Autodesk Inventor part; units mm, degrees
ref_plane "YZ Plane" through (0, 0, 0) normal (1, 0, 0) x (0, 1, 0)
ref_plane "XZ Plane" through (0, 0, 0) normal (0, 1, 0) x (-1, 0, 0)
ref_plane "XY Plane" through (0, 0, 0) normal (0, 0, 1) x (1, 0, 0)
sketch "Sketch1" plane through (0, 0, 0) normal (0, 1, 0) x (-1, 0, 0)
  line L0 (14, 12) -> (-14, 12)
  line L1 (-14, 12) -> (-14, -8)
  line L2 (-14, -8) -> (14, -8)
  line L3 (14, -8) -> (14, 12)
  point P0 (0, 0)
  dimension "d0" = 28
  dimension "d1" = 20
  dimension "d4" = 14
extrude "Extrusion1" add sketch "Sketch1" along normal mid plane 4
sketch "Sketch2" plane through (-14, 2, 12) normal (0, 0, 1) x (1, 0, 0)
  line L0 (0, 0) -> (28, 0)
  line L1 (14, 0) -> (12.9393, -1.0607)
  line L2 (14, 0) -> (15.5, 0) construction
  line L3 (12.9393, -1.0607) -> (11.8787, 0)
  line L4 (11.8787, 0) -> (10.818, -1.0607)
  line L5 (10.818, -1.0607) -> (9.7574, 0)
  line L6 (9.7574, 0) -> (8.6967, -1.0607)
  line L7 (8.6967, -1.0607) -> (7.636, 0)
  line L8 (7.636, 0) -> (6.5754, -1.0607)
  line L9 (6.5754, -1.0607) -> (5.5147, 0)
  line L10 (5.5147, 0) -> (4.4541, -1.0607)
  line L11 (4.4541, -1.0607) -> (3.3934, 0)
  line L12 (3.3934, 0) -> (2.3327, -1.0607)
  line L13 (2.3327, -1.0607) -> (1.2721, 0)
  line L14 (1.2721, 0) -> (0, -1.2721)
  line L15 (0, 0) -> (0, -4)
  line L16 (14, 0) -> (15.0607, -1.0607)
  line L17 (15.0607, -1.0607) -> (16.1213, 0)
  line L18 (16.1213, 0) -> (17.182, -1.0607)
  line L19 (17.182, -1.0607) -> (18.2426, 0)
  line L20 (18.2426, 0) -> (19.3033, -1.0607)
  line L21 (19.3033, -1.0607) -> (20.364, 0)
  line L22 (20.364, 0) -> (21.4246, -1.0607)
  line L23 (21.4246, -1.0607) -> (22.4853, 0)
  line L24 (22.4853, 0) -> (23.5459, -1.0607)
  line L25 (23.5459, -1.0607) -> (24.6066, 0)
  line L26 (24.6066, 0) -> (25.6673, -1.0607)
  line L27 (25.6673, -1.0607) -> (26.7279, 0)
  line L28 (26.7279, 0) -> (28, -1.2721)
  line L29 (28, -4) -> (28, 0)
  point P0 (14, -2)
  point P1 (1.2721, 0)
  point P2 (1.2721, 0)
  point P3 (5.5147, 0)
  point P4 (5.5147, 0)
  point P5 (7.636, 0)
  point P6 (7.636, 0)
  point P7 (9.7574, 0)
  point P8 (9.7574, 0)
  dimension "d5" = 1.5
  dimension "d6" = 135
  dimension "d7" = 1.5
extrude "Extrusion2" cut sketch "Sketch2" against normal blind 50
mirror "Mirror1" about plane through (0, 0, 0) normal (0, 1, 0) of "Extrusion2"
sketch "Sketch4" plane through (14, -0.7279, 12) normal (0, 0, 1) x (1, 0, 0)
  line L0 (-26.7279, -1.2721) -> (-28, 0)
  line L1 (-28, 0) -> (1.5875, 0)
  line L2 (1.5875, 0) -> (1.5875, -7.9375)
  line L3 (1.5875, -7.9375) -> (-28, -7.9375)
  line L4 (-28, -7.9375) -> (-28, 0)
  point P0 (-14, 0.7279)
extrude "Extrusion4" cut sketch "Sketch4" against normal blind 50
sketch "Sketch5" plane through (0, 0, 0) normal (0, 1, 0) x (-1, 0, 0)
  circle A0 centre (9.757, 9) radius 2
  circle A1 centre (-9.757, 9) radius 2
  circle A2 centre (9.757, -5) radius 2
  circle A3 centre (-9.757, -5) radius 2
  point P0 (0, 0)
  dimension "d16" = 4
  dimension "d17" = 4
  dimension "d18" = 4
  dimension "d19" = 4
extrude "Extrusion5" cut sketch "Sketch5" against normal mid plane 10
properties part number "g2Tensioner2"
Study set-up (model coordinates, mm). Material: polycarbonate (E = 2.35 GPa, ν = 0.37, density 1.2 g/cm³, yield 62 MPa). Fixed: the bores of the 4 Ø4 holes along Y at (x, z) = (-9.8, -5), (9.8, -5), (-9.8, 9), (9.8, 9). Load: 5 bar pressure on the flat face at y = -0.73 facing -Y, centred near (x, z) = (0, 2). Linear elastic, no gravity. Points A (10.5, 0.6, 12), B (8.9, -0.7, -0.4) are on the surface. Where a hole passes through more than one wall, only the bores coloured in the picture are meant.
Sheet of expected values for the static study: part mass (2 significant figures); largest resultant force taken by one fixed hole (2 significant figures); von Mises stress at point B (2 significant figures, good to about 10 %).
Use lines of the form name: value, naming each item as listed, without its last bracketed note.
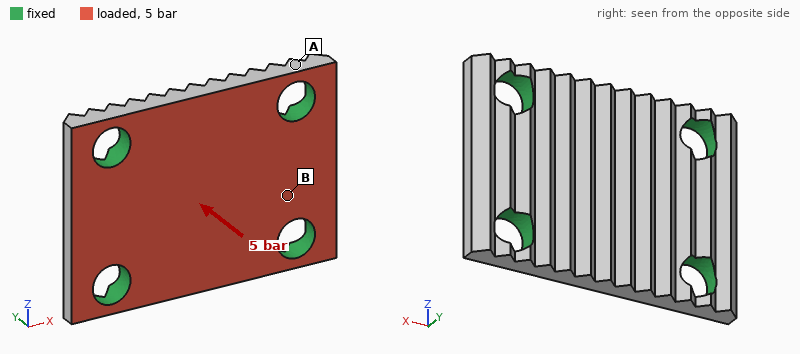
part mass: 1.3 g
largest resultant force taken by one fixed hole: 64 N
von Mises stress at point B: 6.1 MPa
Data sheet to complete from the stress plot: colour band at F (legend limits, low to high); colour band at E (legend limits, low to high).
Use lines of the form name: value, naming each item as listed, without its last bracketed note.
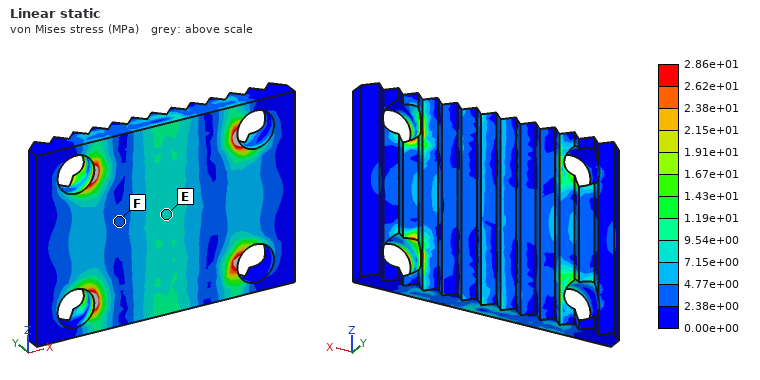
colour band at F: 2.38e+00 to 4.77e+00 MPa
colour band at E: 7.15e+00 to 9.54e+00 MPa
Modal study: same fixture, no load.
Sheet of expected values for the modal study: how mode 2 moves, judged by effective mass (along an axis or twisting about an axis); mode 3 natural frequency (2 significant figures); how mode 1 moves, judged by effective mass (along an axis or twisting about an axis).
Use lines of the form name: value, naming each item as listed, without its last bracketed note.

how mode 2 moves, judged by effective mass: twisting about X
mode 3 natural frequency: 14 kHz
how mode 1 moves, judged by effective mass: along Y
